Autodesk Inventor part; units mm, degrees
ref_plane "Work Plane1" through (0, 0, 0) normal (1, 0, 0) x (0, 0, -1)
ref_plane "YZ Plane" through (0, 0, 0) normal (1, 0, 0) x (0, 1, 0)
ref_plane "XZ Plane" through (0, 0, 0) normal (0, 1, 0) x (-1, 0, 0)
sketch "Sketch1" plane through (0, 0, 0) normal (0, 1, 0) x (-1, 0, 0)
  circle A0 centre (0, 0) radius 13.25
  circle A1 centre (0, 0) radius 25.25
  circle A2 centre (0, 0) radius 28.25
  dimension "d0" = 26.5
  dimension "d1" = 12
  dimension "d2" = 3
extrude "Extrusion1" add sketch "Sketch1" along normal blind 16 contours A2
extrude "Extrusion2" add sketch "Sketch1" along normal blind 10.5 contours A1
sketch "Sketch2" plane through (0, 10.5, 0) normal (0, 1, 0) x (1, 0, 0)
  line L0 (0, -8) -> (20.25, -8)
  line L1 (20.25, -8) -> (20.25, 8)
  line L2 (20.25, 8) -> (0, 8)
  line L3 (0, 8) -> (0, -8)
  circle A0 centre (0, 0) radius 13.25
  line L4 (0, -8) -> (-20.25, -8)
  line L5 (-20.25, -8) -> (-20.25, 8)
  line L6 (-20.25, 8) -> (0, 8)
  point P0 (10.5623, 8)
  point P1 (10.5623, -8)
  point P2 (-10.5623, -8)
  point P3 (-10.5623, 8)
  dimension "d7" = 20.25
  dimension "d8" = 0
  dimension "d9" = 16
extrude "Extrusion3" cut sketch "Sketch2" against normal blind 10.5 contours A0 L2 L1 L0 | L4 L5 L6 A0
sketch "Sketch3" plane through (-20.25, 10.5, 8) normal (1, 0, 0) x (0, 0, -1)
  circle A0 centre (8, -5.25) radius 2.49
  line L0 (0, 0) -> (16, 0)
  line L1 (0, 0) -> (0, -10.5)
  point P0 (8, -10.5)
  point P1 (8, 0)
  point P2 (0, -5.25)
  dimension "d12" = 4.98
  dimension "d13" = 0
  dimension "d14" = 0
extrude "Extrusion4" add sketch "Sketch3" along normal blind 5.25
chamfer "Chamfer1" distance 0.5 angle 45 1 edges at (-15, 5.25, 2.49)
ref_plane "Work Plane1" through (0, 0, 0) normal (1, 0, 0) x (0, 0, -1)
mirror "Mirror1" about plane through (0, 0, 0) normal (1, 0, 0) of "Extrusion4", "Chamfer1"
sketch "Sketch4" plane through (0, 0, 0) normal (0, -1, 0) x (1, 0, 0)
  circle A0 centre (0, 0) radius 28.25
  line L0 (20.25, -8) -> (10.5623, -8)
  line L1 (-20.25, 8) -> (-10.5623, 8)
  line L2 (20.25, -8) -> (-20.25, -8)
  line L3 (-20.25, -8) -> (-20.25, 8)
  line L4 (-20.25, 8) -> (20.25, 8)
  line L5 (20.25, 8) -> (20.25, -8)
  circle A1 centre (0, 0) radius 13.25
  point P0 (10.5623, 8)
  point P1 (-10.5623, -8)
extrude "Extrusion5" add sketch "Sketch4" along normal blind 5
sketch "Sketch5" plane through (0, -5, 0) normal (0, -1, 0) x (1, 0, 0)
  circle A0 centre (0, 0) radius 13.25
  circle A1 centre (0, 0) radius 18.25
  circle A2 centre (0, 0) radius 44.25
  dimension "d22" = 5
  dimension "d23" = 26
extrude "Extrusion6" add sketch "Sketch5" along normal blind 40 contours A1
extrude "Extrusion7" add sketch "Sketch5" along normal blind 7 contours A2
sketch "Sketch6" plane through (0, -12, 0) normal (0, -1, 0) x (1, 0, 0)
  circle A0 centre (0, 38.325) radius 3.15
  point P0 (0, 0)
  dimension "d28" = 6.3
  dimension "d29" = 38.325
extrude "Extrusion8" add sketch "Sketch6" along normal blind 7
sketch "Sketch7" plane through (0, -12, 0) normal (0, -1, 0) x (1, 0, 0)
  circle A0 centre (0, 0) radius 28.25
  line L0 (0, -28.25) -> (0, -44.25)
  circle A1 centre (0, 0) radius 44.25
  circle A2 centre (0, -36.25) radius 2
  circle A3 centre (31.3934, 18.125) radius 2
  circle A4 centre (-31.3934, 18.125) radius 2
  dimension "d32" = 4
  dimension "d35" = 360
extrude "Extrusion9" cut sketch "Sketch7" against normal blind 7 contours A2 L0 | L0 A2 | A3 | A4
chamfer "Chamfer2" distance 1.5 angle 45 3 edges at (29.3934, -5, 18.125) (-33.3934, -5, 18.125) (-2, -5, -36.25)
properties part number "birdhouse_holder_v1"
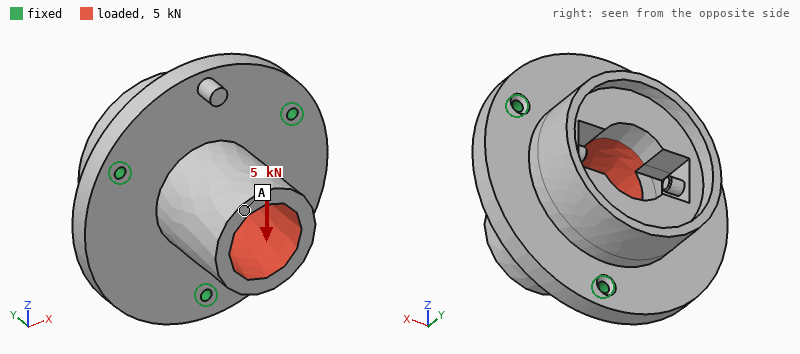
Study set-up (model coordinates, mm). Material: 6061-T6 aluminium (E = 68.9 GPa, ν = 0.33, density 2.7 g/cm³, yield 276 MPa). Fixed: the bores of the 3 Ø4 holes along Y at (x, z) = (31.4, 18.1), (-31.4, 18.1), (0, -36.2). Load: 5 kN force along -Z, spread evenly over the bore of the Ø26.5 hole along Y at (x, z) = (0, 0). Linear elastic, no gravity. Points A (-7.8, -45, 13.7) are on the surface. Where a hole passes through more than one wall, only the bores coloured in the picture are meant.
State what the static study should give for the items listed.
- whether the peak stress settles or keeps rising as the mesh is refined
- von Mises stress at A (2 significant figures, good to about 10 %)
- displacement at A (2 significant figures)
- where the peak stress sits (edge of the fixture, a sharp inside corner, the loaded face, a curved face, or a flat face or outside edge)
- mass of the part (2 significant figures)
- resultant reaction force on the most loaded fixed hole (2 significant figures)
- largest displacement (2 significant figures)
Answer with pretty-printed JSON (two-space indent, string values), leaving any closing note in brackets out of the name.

{
  "whether the peak stress settles or keeps rising as the mesh is refined": "keeps rising",
  "von Mises stress at A": "5.1 MPa",
  "displacement at A": "42 µm",
  "where the peak stress sits": "edge of the fixture",
  "mass of the part": "230 g",
  "resultant reaction force on the most loaded fixed hole": "1.9 kN",
  "largest displacement": "43 µm"
}
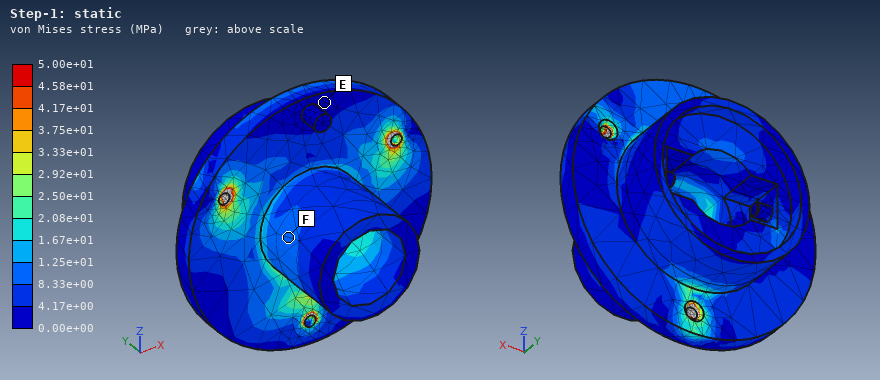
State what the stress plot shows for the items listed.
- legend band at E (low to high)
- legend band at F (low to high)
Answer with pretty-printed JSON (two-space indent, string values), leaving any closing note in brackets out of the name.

{
  "legend band at E": "0.00e+00 to 4.17e+00 MPa",
  "legend band at F": "8.33e+00 to 1.25e+01 MPa"
}
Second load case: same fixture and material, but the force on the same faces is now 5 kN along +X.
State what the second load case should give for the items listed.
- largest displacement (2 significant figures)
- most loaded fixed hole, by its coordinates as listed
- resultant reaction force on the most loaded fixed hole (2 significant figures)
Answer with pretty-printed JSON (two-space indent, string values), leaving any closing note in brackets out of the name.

{
  "largest displacement": "43 µm",
  "most loaded fixed hole, by its coordinates as listed": "(0, -36.2)",
  "resultant reaction force on the most loaded fixed hole": "2.1 kN"
}
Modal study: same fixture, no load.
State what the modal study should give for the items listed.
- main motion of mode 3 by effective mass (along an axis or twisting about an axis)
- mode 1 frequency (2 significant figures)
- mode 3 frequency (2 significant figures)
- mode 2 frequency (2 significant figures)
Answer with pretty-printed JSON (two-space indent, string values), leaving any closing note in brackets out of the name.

{
  "main motion of mode 3 by effective mass": "along Y",
  "mode 1 frequency": "5500 Hz",
  "mode 3 frequency": "6200 Hz",
  "mode 2 frequency": "5600 Hz"
}
